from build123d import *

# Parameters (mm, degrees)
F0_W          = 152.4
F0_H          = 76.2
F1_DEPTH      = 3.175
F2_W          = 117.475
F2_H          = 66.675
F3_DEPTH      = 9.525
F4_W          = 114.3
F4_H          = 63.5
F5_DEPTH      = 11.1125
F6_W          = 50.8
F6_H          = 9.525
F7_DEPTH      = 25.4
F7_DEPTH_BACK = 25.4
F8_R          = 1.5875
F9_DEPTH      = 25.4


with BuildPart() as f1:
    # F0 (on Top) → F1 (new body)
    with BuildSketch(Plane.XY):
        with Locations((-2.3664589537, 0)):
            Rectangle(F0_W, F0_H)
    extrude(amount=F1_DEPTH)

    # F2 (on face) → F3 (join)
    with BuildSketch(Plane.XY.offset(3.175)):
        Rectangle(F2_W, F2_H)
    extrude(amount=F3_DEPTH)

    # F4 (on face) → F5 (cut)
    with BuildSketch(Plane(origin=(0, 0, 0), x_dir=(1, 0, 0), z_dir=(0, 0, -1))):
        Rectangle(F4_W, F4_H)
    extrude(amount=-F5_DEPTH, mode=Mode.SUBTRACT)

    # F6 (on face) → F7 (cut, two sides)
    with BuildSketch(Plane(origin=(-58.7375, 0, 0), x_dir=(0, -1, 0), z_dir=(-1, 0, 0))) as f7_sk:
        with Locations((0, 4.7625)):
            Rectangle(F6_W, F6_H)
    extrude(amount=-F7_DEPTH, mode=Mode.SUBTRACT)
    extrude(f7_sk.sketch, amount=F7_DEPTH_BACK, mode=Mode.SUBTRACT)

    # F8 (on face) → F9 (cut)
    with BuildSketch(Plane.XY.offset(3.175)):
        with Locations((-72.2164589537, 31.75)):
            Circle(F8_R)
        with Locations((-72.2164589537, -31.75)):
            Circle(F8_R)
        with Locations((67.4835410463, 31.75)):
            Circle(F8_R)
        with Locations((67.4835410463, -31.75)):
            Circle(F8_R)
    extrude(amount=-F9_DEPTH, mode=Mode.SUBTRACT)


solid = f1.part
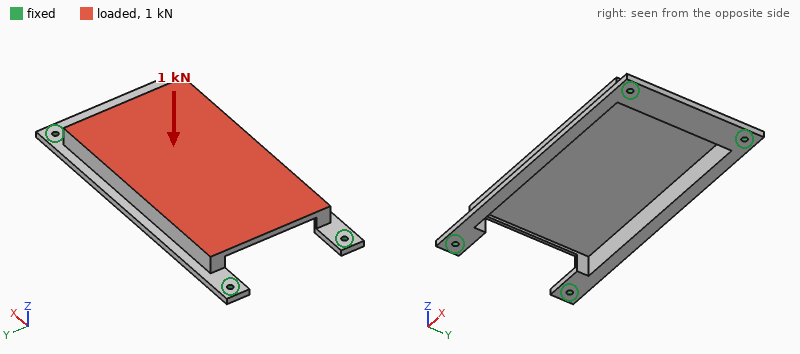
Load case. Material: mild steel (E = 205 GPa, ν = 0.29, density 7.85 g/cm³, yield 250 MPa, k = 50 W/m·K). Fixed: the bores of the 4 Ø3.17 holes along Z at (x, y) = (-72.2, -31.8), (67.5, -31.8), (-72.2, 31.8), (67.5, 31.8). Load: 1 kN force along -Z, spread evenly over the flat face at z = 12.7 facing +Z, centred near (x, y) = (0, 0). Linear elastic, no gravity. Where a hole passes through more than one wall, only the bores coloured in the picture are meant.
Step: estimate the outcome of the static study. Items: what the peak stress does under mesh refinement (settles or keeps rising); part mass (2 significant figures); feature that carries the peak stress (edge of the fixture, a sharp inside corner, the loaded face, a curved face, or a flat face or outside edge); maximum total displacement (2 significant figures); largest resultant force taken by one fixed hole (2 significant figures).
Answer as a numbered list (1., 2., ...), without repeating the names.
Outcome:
1. keeps rising
2. 210 g
3. edge of the fixture
4. 0.17 mm
5. 530 N
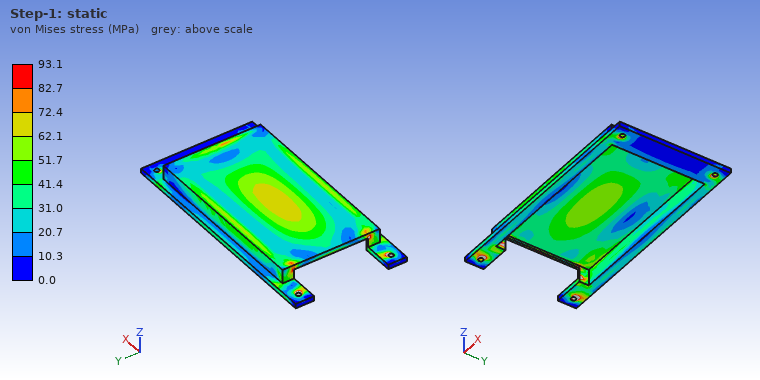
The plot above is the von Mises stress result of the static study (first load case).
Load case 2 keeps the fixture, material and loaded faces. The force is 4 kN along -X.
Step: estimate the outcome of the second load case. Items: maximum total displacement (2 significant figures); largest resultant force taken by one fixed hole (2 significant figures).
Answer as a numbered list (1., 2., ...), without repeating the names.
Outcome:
1. 17 µm
2. 1.1 kN
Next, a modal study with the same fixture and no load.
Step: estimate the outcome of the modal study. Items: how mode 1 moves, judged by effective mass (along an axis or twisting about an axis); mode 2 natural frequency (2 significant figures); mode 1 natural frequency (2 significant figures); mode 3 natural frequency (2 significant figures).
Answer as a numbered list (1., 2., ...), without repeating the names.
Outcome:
1. along Z
2. 2300 Hz
3. 1500 Hz
4. 2500 Hz
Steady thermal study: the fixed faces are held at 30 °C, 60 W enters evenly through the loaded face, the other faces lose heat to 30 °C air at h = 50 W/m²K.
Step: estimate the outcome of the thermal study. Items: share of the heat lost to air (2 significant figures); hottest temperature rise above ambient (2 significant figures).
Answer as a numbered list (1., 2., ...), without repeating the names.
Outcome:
1. 75 %
2. 77 K
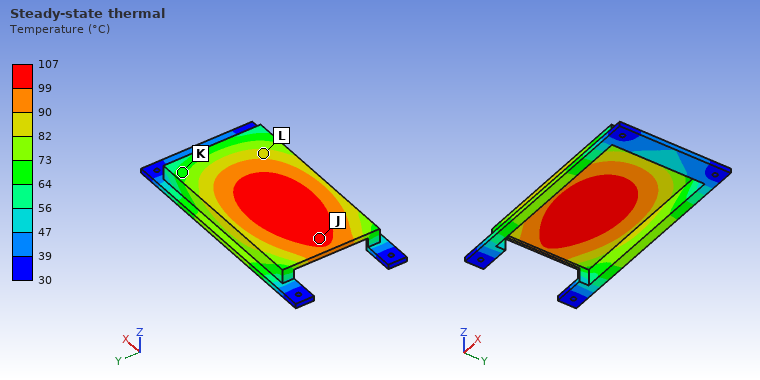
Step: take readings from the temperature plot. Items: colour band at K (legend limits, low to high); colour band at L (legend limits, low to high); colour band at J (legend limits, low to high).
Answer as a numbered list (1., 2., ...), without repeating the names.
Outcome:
1. 64 to 73 °C
2. 82 to 90 °C
3. 99 to 107 °C
